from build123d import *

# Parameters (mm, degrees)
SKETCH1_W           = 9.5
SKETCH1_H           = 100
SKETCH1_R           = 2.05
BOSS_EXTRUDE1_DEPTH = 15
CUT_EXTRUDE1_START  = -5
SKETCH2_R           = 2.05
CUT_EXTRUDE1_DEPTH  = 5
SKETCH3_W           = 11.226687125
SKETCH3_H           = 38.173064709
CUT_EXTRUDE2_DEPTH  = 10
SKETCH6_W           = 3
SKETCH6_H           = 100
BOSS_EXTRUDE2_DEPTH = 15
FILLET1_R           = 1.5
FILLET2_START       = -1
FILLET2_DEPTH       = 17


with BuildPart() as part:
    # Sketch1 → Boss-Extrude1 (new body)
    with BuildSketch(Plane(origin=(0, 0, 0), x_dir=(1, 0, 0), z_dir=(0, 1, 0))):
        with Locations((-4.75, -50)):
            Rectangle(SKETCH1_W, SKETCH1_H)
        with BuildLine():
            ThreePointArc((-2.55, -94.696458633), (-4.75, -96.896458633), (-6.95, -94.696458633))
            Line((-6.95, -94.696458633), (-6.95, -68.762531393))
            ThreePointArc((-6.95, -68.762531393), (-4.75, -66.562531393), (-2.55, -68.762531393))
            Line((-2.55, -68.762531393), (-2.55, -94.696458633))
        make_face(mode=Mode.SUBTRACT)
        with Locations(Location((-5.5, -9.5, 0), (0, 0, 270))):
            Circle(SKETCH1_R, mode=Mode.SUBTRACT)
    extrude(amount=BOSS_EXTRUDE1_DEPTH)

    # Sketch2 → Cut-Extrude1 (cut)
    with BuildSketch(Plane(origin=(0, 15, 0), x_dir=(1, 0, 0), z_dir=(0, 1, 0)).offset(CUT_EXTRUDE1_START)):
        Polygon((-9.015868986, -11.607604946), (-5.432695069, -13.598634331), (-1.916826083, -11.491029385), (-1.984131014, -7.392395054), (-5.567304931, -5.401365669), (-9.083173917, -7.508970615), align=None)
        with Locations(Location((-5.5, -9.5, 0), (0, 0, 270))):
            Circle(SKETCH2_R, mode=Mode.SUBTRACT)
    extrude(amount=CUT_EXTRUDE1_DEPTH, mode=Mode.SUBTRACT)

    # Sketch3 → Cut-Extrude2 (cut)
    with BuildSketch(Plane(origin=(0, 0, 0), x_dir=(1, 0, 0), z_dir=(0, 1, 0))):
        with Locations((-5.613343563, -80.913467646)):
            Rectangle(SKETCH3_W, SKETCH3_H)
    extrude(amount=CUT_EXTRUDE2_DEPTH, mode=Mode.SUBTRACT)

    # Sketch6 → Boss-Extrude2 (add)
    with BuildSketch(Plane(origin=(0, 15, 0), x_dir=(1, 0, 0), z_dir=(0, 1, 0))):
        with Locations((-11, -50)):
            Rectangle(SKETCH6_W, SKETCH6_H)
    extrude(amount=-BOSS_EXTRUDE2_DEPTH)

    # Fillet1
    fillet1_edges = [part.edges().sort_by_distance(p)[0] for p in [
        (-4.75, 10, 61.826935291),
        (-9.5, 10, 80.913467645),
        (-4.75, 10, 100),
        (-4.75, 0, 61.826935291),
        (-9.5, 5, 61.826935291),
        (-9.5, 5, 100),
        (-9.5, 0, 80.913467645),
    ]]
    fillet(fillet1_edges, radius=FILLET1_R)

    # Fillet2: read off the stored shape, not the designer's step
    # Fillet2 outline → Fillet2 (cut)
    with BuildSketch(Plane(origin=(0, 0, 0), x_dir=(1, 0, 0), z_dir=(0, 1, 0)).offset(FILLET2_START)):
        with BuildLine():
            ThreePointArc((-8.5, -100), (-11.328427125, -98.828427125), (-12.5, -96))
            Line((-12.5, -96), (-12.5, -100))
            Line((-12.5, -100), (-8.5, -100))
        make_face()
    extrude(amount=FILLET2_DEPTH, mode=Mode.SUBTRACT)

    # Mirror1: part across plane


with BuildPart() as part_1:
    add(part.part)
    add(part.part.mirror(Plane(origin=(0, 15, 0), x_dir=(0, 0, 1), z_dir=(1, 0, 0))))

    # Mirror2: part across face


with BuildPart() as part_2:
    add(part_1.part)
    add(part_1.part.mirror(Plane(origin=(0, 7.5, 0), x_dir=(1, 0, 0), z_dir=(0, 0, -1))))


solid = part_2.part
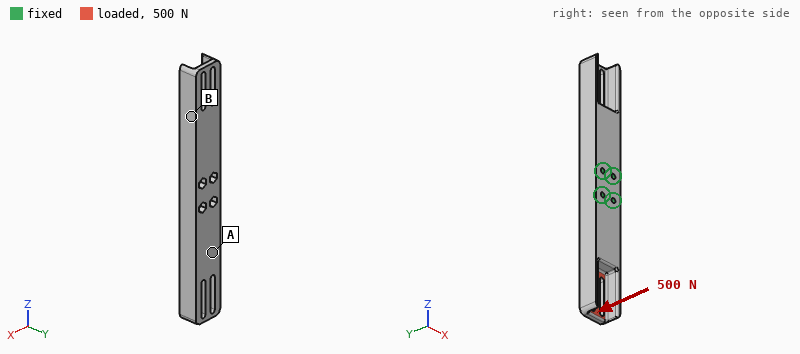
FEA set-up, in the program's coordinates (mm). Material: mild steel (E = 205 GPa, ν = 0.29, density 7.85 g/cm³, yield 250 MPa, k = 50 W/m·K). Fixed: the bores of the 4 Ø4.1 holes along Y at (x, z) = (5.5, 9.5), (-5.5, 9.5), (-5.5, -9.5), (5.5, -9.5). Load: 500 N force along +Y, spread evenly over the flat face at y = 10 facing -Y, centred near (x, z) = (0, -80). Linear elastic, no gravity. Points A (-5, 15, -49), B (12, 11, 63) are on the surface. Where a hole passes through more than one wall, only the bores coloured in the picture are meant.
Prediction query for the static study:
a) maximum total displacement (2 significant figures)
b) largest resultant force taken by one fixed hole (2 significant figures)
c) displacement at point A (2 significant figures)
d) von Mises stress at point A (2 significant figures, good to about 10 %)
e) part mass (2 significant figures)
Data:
81 µm
670 N
23 µm
17 MPa
440 g
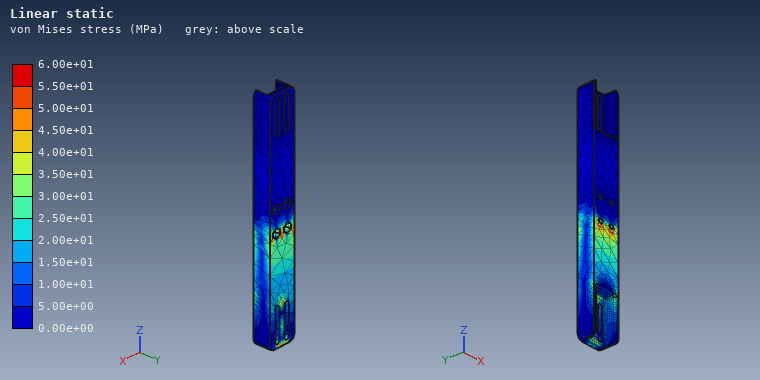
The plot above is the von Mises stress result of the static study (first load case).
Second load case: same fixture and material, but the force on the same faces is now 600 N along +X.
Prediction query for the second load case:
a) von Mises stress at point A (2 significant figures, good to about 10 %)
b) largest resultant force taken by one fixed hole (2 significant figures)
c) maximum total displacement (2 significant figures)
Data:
7.0 MPa
2.3 kN
60 µm
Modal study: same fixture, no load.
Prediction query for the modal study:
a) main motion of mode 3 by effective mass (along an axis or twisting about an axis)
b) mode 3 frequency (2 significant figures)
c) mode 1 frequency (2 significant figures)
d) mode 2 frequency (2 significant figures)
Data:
twisting about Y
2700 Hz
1900 Hz
1900 Hz
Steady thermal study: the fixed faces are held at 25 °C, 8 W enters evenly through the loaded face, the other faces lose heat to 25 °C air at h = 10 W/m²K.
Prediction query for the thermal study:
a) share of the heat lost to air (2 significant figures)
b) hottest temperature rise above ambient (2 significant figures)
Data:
19 %
48 K
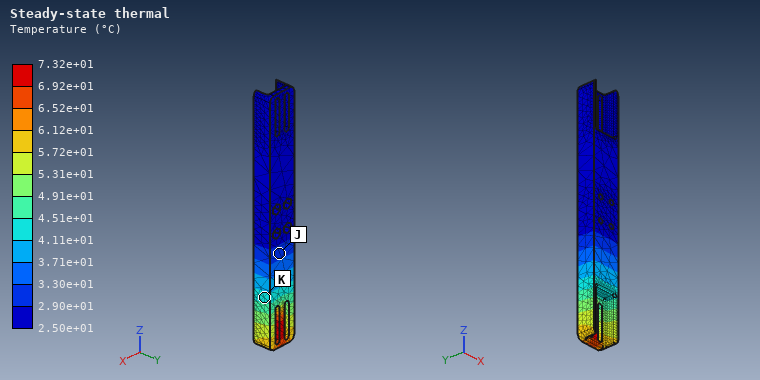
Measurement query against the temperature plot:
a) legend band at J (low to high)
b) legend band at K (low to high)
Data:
2.90e+01 to 3.30e+01 °C
4.11e+01 to 4.51e+01 °C
